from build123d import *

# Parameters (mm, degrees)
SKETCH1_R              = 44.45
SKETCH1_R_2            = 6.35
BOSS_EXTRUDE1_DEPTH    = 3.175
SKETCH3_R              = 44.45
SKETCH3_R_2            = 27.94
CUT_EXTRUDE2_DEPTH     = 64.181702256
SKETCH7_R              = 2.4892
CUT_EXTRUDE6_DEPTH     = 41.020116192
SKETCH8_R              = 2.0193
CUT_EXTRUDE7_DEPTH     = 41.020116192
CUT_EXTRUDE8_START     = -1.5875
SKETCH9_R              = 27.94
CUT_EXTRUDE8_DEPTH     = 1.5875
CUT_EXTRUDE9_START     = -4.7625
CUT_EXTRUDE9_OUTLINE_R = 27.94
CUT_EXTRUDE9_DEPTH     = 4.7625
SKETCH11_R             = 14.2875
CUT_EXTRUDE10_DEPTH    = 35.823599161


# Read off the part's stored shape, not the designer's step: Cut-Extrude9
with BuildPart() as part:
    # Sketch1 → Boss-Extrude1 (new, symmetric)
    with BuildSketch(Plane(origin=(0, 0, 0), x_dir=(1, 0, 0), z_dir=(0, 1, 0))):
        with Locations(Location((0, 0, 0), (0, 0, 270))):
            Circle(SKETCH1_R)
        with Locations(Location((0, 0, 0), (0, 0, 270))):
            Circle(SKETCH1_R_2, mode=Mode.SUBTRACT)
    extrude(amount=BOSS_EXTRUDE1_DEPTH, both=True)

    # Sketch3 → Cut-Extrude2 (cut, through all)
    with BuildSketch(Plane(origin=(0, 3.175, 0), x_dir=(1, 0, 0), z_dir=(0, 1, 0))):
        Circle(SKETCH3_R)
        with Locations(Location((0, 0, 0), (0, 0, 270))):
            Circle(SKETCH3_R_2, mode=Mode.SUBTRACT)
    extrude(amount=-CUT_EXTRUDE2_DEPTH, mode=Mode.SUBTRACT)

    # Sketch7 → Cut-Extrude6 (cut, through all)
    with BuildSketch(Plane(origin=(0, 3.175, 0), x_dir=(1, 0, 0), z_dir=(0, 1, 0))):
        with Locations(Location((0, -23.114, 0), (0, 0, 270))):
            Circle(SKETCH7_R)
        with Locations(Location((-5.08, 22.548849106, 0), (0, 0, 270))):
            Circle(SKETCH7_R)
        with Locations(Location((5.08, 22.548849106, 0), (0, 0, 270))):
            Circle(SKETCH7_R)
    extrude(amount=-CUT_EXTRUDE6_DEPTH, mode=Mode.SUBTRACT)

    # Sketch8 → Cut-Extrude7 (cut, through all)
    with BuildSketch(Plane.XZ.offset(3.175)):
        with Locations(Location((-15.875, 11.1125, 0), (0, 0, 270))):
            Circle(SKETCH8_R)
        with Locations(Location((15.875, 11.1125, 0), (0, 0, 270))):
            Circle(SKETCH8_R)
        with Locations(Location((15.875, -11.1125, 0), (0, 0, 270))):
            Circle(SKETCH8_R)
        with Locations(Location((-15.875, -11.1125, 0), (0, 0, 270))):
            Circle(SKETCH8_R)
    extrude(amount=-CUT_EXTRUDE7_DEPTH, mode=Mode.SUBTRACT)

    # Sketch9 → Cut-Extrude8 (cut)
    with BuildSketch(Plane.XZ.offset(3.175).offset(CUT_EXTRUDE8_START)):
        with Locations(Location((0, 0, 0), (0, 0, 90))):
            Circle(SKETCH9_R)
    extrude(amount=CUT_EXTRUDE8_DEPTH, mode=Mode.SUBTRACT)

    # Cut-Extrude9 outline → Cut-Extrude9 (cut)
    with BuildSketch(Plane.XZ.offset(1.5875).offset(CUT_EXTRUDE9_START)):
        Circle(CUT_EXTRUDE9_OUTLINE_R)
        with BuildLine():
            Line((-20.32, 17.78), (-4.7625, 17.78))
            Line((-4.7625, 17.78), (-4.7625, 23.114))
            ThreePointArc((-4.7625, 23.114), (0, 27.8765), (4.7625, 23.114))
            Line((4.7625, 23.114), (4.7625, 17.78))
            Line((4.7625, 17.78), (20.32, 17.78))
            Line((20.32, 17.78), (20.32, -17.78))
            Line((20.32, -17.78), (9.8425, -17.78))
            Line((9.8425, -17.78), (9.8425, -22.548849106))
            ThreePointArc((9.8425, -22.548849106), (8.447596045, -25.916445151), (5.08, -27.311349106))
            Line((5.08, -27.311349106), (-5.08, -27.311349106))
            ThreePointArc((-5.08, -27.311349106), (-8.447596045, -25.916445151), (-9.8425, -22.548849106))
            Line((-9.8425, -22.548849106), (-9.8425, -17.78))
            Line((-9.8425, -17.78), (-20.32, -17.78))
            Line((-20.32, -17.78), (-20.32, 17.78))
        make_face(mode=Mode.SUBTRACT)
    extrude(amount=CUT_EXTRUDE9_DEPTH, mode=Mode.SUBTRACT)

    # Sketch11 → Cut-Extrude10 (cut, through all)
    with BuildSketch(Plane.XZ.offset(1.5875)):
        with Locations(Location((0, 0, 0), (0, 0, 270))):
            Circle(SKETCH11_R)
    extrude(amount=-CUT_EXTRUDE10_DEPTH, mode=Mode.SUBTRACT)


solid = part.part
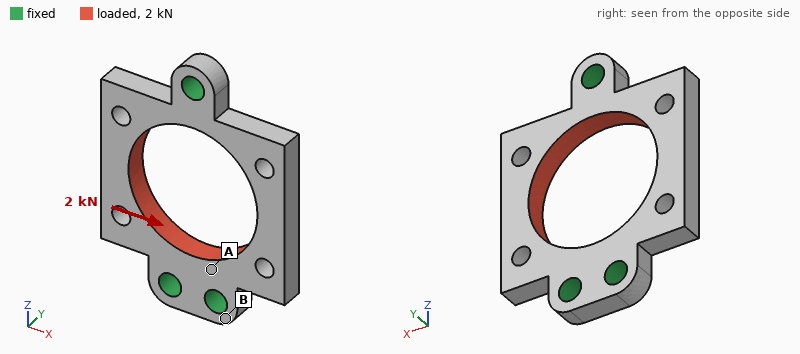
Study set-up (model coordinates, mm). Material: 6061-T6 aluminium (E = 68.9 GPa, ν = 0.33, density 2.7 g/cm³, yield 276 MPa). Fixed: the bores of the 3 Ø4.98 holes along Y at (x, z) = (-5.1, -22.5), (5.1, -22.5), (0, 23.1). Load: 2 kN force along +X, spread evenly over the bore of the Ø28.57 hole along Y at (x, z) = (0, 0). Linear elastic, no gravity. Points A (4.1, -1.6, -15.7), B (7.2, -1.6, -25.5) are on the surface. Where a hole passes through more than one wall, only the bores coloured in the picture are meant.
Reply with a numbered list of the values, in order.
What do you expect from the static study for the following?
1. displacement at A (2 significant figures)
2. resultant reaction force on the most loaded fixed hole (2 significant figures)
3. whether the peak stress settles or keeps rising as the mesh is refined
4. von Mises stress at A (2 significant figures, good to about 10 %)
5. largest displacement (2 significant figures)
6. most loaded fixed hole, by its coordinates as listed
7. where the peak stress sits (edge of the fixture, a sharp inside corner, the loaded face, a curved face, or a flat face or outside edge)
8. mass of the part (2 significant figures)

1. 2.3 µm
2. 1.0 kN
3. keeps rising
4. 17 MPa
5. 11 µm
6. (0, 23.1)
7. edge of the fixture
8. 12 g
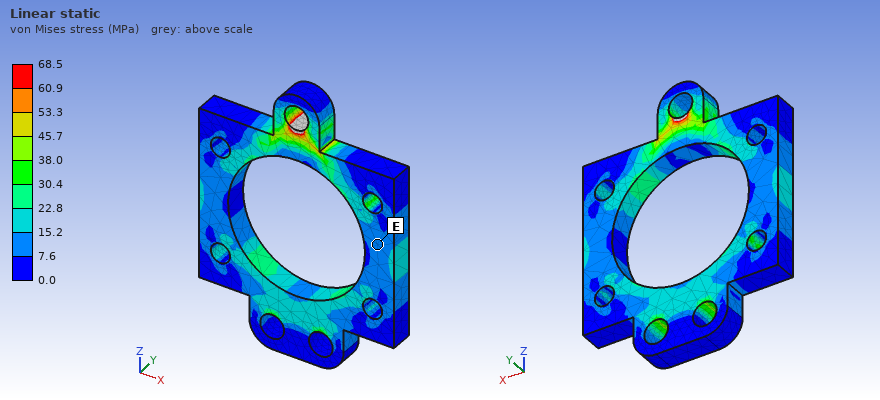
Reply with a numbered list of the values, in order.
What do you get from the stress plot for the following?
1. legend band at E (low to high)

1. 7.6 to 15.2 MPa
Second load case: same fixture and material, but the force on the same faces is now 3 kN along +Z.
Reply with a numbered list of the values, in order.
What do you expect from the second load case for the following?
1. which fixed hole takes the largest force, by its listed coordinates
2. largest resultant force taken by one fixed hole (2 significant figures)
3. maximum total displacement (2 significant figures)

1. (0, 23.1)
2. 1.2 kN
3. 16 µm
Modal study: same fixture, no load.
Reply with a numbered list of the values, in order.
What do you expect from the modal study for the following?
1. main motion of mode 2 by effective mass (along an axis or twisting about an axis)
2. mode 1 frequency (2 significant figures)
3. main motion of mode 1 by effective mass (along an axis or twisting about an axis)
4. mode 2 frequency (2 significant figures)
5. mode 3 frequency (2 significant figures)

1. along Y
2. 5600 Hz
3. twisting about Z
4. 6300 Hz
5. 13 kHz
